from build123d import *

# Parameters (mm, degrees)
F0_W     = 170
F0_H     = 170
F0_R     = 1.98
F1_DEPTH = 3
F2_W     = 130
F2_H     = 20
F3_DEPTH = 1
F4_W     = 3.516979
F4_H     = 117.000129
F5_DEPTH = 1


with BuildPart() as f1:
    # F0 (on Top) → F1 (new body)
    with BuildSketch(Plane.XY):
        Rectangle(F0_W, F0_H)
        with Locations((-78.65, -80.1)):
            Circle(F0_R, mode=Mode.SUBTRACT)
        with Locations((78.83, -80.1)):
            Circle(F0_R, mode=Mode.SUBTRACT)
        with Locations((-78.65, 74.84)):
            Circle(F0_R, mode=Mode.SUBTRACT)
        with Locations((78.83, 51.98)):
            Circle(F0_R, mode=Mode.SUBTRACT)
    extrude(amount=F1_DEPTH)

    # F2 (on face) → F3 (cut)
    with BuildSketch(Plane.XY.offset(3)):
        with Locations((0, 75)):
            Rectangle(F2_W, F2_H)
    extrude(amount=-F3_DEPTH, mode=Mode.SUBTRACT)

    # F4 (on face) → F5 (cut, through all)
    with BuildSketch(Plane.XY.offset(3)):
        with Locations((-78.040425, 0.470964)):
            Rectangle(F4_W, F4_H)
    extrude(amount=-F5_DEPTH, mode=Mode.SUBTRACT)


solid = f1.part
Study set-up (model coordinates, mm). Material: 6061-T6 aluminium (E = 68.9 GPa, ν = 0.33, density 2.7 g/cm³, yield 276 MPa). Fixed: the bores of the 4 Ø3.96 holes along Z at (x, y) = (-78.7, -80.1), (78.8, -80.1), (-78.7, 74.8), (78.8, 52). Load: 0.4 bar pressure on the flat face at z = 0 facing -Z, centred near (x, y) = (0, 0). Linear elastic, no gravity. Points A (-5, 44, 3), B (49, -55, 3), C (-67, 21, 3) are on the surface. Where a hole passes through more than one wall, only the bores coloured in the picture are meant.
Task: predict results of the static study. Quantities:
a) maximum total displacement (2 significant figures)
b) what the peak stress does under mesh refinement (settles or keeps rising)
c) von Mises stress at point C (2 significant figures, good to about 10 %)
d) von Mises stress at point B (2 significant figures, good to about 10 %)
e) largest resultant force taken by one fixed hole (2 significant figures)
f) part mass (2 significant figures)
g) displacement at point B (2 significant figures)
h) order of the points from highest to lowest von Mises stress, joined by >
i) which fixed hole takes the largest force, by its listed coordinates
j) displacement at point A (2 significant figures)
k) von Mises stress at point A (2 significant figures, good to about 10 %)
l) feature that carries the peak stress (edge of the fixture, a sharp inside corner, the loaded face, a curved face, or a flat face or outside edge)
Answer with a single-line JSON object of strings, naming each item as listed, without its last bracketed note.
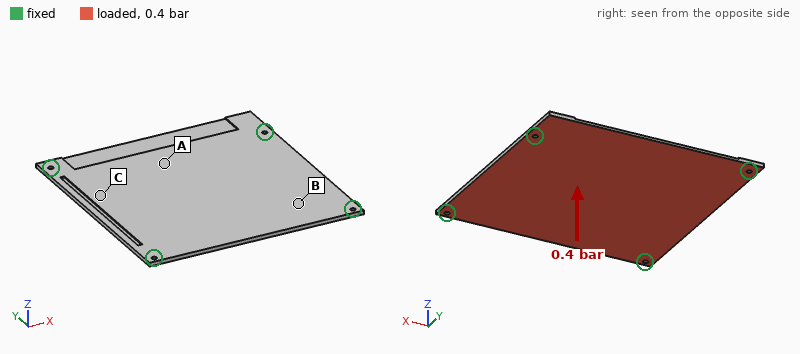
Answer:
{"maximum total displacement": "1.2 mm", "what the peak stress does under mesh refinement": "keeps rising", "von Mises stress at point C": "33 MPa", "von Mises stress at point B": "14 MPa", "largest resultant force taken by one fixed hole": "380 N", "part mass": "230 g", "displacement at point B": "0.53 mm", "order of the points from highest to lowest von Mises stress, joined by >": "A > C > B", "which fixed hole takes the largest force, by its listed coordinates": "(78.8, 52)", "displacement at point A": "0.97 mm", "von Mises stress at point A": "43 MPa", "feature that carries the peak stress": "edge of the fixture"}
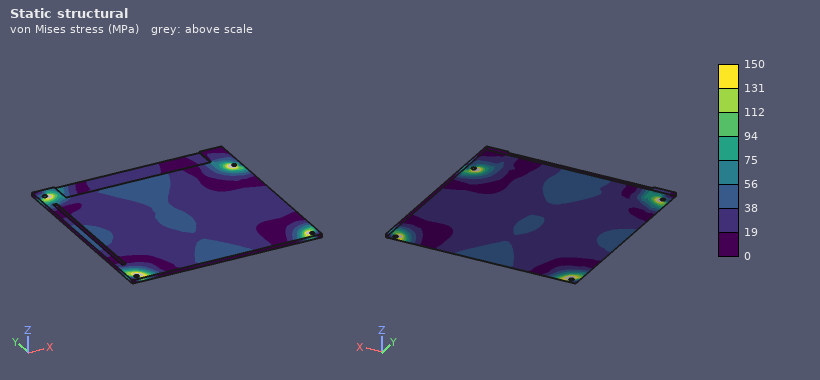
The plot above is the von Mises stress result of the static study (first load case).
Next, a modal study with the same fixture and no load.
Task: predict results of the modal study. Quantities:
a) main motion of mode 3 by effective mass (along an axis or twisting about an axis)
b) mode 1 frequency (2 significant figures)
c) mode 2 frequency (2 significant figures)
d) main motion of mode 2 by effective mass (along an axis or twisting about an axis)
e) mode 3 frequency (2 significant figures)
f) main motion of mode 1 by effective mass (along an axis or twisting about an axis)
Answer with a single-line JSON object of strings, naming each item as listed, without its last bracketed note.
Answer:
{"main motion of mode 3 by effective mass": "twisting about Y", "mode 1 frequency": "390 Hz", "mode 2 frequency": "640 Hz", "main motion of mode 2 by effective mass": "twisting about X", "mode 3 frequency": "720 Hz", "main motion of mode 1 by effective mass": "along Z"}
